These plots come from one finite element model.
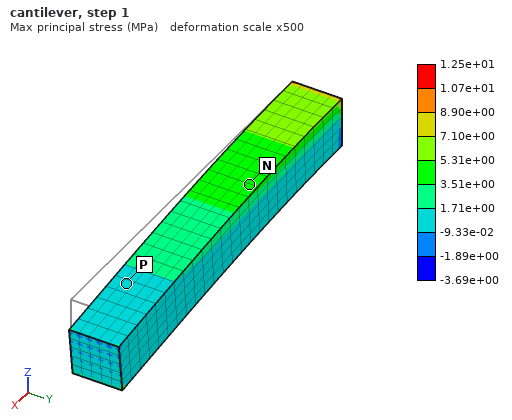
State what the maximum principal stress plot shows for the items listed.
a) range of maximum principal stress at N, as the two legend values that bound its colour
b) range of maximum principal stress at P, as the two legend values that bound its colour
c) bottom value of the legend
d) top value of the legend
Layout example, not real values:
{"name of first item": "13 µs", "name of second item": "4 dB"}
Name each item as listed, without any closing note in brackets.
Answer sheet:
{"range of maximum principal stress at N, as the two legend values that bound its colour": "3.51e+00 to 5.31e+00 MPa", "range of maximum principal stress at P, as the two legend values that bound its colour": "-9.33e-02 to 1.71e+00 MPa", "bottom value of the legend": "-3.69e+00 MPa", "top value of the legend": "1.25e+01 MPa"}
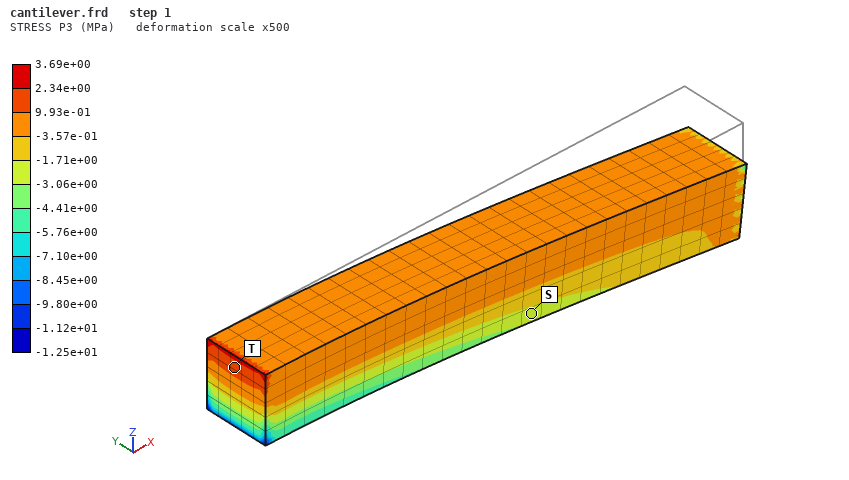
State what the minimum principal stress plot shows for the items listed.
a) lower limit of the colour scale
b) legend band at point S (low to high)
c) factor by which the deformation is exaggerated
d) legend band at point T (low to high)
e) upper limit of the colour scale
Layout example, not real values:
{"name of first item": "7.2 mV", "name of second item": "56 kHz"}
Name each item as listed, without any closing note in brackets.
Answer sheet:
{"lower limit of the colour scale": "-1.25e+01 MPa", "legend band at point S": "-3.06e+00 to -1.71e+00 MPa", "factor by which the deformation is exaggerated": "500", "legend band at point T": "9.93e-01 to 2.34e+00 MPa", "upper limit of the colour scale": "3.69e+00 MPa"}
